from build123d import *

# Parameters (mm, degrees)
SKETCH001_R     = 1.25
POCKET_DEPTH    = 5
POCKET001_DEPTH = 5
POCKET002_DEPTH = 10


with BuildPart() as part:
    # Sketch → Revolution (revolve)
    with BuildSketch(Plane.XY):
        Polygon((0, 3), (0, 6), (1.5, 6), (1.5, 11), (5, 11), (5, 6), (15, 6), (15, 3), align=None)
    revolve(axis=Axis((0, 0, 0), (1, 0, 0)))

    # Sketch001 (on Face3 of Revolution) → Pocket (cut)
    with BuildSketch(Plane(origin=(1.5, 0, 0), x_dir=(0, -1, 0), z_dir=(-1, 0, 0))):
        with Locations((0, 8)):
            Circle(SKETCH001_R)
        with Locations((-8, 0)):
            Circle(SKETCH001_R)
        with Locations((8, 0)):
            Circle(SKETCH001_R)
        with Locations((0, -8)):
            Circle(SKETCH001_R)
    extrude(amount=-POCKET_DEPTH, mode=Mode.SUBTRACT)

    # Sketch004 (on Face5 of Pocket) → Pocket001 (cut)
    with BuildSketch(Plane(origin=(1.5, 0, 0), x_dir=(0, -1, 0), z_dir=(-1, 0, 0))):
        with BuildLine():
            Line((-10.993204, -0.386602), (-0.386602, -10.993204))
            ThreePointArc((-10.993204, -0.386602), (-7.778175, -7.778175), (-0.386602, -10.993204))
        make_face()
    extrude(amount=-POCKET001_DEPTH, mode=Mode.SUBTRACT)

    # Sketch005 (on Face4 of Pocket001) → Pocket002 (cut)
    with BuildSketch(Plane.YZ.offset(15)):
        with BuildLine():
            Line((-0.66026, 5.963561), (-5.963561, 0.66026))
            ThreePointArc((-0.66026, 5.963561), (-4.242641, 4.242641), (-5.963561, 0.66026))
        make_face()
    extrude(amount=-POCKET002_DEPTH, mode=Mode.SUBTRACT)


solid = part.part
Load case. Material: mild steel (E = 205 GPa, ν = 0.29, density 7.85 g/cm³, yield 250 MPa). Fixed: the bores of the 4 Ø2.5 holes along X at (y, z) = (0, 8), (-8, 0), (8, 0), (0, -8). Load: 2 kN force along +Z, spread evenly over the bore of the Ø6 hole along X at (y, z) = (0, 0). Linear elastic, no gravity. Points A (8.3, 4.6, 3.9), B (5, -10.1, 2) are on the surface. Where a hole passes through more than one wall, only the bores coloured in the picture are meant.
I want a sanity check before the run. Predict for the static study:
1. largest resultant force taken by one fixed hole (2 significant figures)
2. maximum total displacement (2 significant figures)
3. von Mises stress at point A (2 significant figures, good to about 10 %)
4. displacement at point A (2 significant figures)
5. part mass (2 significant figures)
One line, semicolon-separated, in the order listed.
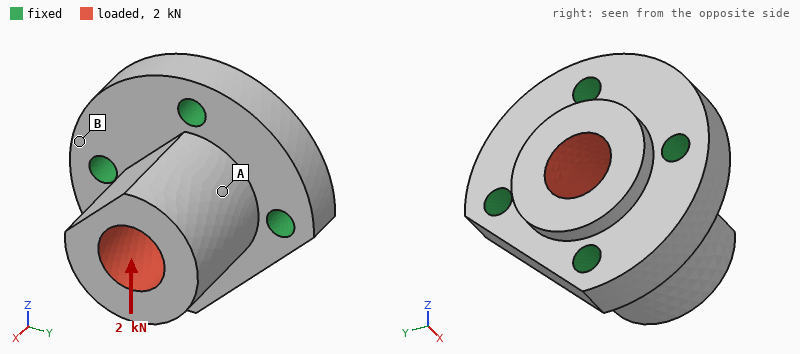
860 N; 5.4 µm; 20 MPa; 2.3 µm; 15 g
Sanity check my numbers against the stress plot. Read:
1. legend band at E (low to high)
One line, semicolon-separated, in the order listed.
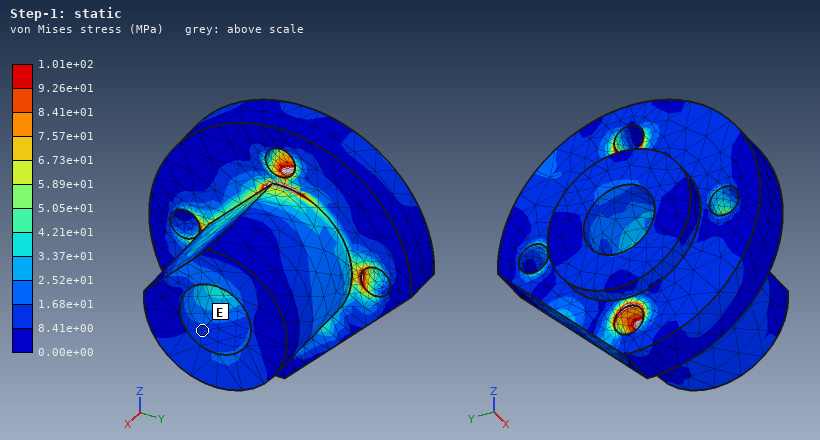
8.41e+00 to 1.68e+01 MPa
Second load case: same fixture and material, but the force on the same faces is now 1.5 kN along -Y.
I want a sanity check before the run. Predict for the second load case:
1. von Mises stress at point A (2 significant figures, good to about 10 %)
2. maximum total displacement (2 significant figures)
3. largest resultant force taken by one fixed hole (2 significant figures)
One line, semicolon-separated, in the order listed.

18 MPa; 4.1 µm; 650 N
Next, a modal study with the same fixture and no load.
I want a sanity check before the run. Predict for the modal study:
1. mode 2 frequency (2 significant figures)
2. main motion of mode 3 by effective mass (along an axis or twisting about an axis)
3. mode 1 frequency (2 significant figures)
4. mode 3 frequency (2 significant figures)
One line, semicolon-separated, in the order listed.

38 kHz; along X; 37 kHz; 66 kHz
